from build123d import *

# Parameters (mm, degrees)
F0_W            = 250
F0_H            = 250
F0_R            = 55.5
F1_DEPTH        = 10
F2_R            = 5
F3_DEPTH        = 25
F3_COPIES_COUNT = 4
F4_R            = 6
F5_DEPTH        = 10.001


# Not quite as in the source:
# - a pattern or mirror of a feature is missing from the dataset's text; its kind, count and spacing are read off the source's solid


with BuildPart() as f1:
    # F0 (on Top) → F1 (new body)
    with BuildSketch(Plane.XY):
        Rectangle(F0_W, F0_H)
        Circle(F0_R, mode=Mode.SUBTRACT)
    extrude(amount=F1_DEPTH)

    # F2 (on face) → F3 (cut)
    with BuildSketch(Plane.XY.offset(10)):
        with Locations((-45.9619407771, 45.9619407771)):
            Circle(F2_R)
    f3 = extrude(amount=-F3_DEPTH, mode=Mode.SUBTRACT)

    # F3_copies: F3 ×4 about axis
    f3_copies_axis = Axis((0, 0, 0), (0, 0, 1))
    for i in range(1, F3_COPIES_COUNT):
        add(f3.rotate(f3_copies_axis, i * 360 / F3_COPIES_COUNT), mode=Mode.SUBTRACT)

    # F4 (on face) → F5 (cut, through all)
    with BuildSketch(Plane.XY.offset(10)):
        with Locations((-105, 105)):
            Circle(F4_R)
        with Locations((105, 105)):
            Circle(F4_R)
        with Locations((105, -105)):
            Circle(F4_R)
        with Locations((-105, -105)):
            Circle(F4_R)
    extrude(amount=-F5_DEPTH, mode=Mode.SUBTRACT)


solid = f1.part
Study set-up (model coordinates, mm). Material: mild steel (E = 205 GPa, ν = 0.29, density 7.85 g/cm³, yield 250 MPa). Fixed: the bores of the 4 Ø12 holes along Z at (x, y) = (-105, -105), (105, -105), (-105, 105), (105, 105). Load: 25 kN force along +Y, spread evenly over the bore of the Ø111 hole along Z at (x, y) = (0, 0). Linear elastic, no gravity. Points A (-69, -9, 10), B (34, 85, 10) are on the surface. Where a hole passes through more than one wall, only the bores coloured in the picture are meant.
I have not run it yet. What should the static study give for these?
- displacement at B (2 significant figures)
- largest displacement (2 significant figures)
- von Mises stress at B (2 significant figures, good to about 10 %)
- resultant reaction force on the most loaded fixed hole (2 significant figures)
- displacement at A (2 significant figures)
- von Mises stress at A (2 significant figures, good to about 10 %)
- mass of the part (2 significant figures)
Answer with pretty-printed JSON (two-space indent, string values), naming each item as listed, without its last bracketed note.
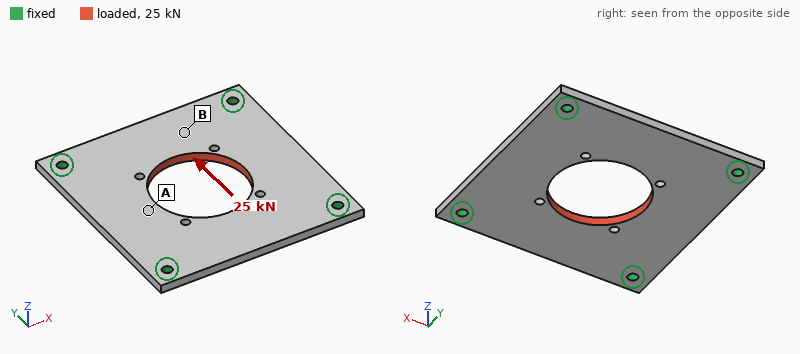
{
  "displacement at B": "7.6 µm",
  "largest displacement": "9.8 µm",
  "von Mises stress at B": "7.6 MPa",
  "resultant reaction force on the most loaded fixed hole": "6.8 kN",
  "displacement at A": "5.3 µm",
  "von Mises stress at A": "13 MPa",
  "mass of the part": "4.1 kg"
}
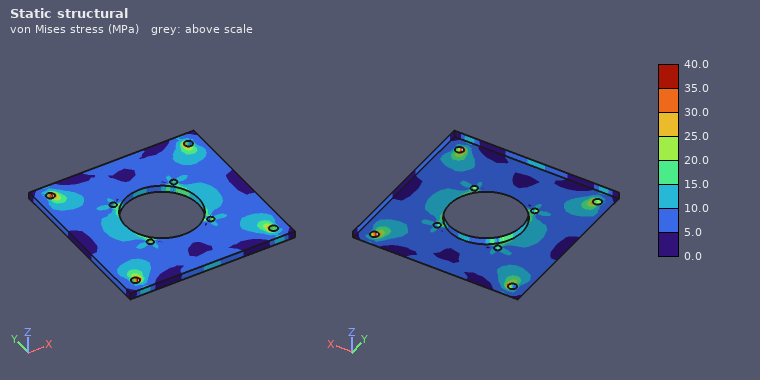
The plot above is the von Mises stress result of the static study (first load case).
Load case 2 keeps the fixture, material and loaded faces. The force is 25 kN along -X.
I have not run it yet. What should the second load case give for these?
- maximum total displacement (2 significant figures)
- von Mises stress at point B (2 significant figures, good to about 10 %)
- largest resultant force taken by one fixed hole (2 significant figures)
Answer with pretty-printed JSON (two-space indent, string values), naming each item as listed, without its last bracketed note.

{
  "maximum total displacement": "9.8 µm",
  "von Mises stress at point B": "8.7 MPa",
  "largest resultant force taken by one fixed hole": "6.8 kN"
}
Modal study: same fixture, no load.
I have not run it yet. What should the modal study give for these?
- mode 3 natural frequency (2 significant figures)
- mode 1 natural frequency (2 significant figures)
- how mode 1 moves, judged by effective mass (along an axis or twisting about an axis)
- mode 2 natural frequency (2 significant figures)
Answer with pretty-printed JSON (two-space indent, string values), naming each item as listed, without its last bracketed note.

{
  "mode 3 natural frequency": "1300 Hz",
  "mode 1 natural frequency": "880 Hz",
  "how mode 1 moves, judged by effective mass": "along Z",
  "mode 2 natural frequency": "1300 Hz"
}
